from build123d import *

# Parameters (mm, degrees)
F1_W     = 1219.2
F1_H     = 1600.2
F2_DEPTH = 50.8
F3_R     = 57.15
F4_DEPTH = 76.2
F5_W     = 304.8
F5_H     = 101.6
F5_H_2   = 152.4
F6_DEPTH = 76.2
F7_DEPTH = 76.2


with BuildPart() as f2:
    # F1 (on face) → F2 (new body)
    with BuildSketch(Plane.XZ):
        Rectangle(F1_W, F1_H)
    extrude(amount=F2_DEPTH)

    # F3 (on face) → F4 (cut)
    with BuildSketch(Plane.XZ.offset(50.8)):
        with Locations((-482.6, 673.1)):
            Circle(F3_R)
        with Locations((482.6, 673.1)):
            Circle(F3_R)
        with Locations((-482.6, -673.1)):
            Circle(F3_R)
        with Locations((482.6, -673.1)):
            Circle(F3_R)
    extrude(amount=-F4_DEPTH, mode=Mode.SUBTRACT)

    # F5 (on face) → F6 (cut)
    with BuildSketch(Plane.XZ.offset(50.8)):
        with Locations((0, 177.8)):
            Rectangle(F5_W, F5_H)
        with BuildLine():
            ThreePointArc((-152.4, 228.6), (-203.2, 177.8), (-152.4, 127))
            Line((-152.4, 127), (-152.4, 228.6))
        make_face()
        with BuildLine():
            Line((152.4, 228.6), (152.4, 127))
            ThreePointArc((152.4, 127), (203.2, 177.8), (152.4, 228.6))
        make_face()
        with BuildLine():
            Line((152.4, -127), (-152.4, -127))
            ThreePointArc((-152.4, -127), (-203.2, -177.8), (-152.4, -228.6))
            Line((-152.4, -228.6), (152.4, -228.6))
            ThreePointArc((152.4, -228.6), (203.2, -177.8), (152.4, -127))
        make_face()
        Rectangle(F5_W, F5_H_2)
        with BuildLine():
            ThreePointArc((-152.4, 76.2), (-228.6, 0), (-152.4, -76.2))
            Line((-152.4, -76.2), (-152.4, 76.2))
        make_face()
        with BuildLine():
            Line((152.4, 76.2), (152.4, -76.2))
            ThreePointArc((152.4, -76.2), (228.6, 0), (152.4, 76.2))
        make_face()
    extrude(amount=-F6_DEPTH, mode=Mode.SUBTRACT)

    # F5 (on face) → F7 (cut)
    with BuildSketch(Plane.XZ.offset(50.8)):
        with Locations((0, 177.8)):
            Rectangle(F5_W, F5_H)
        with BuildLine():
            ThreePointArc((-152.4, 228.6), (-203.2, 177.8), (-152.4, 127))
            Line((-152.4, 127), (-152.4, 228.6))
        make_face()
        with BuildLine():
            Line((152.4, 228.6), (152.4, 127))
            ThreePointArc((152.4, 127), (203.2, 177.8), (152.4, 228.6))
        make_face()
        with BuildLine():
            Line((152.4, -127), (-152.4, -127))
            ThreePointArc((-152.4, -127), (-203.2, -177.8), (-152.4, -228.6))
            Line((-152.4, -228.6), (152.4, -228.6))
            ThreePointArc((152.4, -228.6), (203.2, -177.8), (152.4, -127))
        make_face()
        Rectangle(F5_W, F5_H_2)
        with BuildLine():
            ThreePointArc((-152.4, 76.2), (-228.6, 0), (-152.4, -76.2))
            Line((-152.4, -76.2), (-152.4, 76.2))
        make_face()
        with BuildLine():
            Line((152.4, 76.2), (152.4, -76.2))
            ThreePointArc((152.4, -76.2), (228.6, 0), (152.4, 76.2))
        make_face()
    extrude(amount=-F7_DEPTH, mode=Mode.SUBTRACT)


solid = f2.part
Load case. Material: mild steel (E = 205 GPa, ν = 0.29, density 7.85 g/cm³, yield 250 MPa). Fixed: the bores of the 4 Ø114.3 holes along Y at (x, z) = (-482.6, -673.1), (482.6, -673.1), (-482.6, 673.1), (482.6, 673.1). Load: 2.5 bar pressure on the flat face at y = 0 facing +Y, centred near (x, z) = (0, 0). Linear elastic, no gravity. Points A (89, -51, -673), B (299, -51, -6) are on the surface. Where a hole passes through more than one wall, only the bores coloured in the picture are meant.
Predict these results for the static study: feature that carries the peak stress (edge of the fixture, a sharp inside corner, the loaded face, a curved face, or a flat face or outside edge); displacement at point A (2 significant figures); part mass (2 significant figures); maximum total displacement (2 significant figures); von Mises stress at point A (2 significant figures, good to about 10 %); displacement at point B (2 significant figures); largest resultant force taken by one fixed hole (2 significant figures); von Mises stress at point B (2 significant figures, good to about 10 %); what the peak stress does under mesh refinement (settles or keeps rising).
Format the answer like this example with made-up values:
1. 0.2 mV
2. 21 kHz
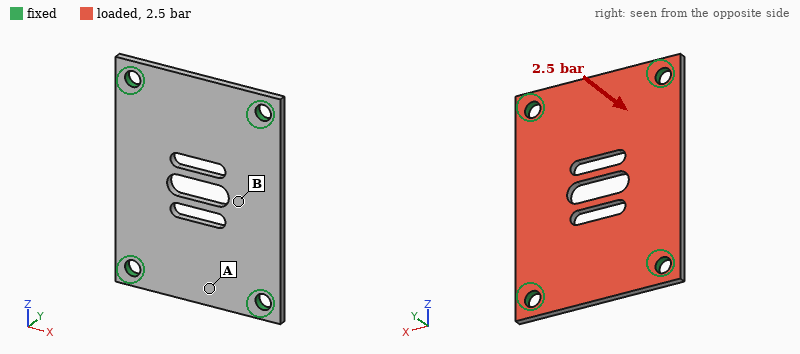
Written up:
1. edge of the fixture
2. 0.24 mm
3. 700 kg
4. 1.4 mm
5. 25 MPa
6. 1.2 mm
7. 110 kN
8. 52 MPa
9. keeps rising
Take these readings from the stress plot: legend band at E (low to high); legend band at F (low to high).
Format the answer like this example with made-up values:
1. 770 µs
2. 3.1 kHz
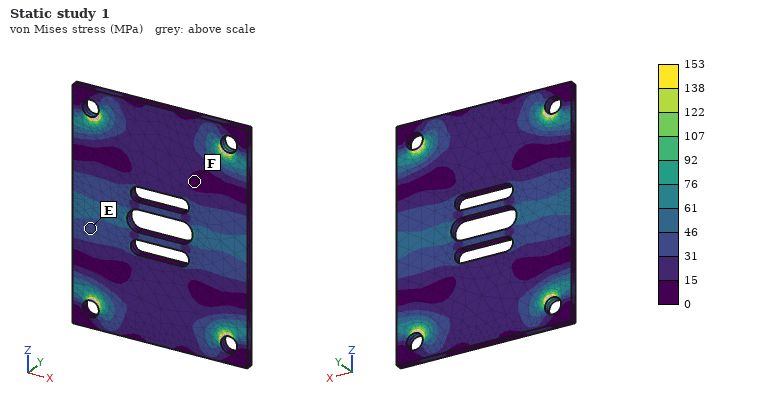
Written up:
1. 31 to 46 MPa
2. 0 to 15 MPa
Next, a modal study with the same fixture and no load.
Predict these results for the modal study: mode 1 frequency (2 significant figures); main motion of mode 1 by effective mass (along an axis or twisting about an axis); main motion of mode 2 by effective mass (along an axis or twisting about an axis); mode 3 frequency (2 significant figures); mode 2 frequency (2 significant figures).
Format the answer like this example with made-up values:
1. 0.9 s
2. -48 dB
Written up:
1. 140 Hz
2. along Y
3. twisting about Z
4. 270 Hz
5. 190 Hz
